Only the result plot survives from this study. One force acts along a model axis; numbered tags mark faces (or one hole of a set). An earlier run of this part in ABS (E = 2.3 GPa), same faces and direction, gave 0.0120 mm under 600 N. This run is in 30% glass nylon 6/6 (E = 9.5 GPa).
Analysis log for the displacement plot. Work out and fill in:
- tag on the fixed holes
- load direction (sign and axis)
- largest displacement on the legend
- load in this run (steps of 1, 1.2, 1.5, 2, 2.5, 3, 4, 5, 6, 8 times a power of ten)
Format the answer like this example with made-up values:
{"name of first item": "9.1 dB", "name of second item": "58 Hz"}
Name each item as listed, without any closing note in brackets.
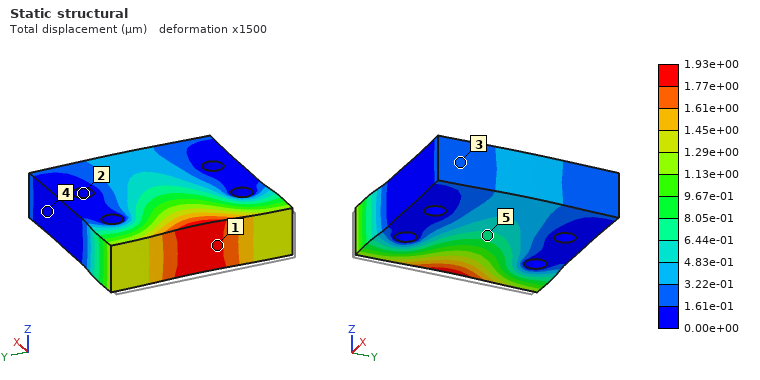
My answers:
{"tag on the fixed holes": "2", "load direction": "+X", "largest displacement on the legend": "1.93e+00 µm", "load in this run": "400 N"}
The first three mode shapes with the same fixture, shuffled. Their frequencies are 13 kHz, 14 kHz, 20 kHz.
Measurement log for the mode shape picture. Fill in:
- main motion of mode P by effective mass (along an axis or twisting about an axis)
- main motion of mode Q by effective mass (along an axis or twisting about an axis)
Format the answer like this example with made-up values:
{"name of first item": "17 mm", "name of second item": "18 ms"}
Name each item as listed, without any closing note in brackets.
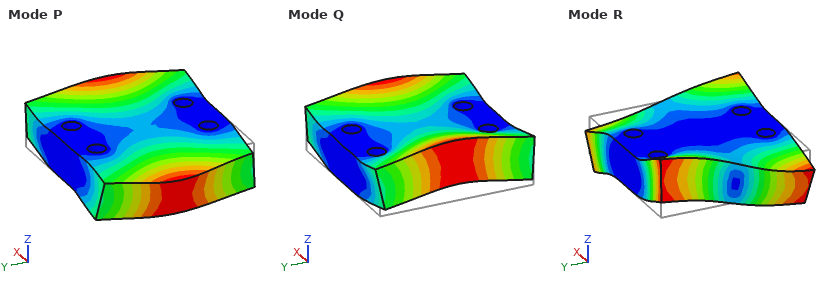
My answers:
{"main motion of mode P by effective mass": "twisting about Y", "main motion of mode Q by effective mass": "along Z"}
